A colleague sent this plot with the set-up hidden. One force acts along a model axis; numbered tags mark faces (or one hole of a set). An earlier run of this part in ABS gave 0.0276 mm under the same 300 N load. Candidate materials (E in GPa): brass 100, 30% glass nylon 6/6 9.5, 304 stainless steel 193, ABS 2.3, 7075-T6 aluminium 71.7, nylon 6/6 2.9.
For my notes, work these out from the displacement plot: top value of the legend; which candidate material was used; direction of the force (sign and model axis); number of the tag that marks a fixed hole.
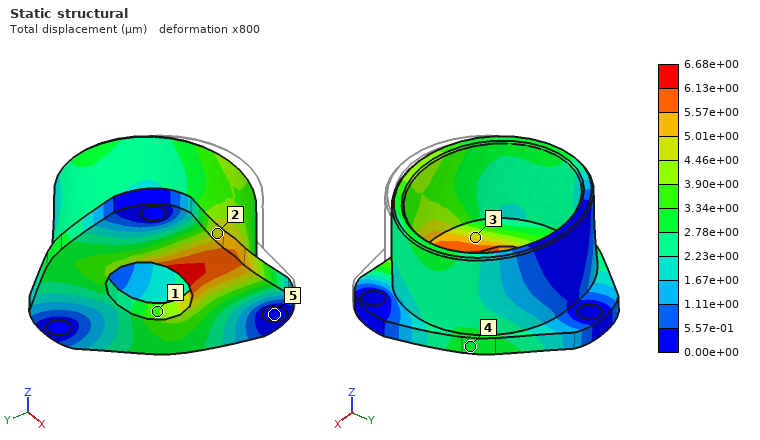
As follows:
6.68e+00 µm
30% glass nylon 6/6
+Y
5
